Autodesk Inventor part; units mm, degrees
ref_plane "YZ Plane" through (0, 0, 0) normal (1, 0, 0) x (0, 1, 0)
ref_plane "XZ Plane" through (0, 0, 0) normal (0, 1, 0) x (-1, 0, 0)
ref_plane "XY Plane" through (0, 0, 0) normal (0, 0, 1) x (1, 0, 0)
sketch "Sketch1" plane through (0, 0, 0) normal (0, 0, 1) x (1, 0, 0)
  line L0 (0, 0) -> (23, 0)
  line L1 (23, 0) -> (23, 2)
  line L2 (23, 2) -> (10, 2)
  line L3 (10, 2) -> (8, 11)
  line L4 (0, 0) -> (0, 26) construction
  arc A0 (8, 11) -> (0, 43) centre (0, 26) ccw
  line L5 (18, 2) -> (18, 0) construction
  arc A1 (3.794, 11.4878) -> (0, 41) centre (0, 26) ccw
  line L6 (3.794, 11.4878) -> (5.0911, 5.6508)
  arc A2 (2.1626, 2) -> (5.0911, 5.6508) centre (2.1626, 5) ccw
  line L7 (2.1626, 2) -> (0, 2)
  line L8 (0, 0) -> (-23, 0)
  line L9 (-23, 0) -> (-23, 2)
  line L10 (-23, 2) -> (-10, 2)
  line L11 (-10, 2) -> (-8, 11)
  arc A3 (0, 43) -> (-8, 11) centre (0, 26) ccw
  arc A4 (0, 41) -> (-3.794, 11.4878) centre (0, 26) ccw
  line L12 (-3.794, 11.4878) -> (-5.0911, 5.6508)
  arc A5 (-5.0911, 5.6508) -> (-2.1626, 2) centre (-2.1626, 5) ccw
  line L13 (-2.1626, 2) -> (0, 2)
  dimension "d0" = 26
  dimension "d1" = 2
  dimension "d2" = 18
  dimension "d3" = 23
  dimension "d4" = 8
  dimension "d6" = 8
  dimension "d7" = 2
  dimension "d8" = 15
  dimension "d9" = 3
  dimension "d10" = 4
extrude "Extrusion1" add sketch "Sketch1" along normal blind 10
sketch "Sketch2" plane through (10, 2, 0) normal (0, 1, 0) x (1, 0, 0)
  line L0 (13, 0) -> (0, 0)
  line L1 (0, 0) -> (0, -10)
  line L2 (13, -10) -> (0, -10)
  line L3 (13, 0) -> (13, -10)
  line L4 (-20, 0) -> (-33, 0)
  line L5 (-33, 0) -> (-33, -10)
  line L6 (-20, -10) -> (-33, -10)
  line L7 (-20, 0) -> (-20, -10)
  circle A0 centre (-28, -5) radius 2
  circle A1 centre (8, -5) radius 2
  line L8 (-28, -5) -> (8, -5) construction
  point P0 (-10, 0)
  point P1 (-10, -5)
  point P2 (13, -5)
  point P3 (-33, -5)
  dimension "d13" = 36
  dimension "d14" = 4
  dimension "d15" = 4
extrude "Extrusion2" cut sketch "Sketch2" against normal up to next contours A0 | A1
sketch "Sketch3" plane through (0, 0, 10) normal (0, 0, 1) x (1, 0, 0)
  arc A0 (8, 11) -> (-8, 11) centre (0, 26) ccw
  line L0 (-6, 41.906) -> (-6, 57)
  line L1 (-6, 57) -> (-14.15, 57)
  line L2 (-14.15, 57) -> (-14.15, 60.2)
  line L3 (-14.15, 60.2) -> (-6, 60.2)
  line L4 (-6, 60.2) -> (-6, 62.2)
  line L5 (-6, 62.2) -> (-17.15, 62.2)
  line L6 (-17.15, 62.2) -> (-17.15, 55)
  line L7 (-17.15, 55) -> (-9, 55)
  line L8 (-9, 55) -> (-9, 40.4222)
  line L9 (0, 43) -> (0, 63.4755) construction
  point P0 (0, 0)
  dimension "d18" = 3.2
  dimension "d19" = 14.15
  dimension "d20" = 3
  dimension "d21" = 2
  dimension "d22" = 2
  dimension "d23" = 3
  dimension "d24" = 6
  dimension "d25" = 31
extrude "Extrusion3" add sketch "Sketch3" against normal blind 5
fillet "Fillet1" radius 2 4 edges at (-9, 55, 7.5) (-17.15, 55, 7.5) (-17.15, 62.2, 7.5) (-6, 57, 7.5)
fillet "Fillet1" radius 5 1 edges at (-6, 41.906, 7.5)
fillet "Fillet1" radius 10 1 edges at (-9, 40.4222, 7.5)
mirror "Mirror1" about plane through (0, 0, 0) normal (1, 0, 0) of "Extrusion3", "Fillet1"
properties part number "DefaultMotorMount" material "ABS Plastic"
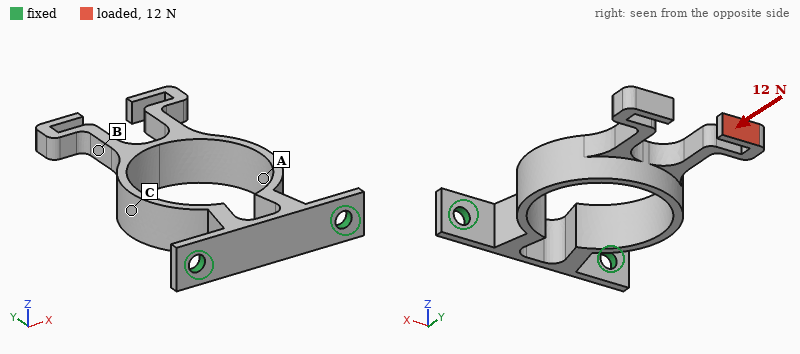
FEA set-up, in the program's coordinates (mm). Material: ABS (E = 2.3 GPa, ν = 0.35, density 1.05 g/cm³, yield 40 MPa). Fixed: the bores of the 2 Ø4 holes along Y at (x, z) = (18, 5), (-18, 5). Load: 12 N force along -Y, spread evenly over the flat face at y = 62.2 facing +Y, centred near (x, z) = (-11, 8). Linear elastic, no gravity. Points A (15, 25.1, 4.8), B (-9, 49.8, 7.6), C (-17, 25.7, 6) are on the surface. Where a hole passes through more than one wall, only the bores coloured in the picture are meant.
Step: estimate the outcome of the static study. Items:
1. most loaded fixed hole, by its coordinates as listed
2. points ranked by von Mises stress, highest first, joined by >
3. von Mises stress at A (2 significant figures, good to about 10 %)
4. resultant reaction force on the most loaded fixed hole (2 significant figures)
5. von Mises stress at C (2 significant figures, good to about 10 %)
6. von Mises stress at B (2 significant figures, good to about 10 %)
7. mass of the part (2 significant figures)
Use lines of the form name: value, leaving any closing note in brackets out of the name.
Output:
most loaded fixed hole, by its coordinates as listed: (-18, 5)
points ranked by von Mises stress, highest first, joined by >: B > C > A
von Mises stress at A: 1.4 MPa
resultant reaction force on the most loaded fixed hole: 11 N
von Mises stress at C: 3.6 MPa
von Mises stress at B: 5.7 MPa
mass of the part: 4.7 g
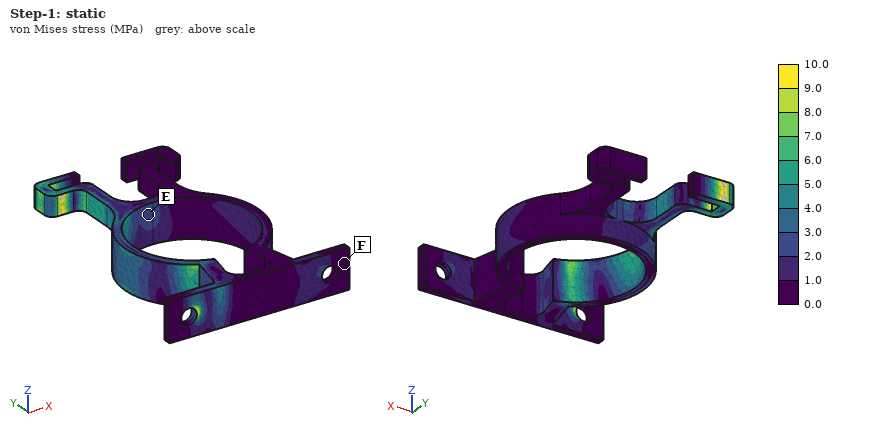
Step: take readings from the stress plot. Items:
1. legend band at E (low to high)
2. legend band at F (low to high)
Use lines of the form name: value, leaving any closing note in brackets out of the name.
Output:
legend band at E: 2.0 to 3.0 MPa
legend band at F: 0.0 to 1.0 MPa
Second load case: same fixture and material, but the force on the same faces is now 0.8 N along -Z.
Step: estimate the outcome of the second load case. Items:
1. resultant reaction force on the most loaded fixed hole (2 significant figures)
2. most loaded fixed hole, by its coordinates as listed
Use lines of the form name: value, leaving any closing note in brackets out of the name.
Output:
resultant reaction force on the most loaded fixed hole: 0.69 N
most loaded fixed hole, by its coordinates as listed: (-18, 5)
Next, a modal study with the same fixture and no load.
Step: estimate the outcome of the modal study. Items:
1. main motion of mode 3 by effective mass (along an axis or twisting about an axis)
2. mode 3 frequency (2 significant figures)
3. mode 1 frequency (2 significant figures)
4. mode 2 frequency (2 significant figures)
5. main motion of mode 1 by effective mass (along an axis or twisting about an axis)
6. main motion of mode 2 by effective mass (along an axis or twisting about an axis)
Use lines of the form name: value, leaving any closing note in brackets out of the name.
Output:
main motion of mode 3 by effective mass: twisting about Y
mode 3 frequency: 640 Hz
mode 1 frequency: 170 Hz
mode 2 frequency: 260 Hz
main motion of mode 1 by effective mass: along Z
main motion of mode 2 by effective mass: along X
